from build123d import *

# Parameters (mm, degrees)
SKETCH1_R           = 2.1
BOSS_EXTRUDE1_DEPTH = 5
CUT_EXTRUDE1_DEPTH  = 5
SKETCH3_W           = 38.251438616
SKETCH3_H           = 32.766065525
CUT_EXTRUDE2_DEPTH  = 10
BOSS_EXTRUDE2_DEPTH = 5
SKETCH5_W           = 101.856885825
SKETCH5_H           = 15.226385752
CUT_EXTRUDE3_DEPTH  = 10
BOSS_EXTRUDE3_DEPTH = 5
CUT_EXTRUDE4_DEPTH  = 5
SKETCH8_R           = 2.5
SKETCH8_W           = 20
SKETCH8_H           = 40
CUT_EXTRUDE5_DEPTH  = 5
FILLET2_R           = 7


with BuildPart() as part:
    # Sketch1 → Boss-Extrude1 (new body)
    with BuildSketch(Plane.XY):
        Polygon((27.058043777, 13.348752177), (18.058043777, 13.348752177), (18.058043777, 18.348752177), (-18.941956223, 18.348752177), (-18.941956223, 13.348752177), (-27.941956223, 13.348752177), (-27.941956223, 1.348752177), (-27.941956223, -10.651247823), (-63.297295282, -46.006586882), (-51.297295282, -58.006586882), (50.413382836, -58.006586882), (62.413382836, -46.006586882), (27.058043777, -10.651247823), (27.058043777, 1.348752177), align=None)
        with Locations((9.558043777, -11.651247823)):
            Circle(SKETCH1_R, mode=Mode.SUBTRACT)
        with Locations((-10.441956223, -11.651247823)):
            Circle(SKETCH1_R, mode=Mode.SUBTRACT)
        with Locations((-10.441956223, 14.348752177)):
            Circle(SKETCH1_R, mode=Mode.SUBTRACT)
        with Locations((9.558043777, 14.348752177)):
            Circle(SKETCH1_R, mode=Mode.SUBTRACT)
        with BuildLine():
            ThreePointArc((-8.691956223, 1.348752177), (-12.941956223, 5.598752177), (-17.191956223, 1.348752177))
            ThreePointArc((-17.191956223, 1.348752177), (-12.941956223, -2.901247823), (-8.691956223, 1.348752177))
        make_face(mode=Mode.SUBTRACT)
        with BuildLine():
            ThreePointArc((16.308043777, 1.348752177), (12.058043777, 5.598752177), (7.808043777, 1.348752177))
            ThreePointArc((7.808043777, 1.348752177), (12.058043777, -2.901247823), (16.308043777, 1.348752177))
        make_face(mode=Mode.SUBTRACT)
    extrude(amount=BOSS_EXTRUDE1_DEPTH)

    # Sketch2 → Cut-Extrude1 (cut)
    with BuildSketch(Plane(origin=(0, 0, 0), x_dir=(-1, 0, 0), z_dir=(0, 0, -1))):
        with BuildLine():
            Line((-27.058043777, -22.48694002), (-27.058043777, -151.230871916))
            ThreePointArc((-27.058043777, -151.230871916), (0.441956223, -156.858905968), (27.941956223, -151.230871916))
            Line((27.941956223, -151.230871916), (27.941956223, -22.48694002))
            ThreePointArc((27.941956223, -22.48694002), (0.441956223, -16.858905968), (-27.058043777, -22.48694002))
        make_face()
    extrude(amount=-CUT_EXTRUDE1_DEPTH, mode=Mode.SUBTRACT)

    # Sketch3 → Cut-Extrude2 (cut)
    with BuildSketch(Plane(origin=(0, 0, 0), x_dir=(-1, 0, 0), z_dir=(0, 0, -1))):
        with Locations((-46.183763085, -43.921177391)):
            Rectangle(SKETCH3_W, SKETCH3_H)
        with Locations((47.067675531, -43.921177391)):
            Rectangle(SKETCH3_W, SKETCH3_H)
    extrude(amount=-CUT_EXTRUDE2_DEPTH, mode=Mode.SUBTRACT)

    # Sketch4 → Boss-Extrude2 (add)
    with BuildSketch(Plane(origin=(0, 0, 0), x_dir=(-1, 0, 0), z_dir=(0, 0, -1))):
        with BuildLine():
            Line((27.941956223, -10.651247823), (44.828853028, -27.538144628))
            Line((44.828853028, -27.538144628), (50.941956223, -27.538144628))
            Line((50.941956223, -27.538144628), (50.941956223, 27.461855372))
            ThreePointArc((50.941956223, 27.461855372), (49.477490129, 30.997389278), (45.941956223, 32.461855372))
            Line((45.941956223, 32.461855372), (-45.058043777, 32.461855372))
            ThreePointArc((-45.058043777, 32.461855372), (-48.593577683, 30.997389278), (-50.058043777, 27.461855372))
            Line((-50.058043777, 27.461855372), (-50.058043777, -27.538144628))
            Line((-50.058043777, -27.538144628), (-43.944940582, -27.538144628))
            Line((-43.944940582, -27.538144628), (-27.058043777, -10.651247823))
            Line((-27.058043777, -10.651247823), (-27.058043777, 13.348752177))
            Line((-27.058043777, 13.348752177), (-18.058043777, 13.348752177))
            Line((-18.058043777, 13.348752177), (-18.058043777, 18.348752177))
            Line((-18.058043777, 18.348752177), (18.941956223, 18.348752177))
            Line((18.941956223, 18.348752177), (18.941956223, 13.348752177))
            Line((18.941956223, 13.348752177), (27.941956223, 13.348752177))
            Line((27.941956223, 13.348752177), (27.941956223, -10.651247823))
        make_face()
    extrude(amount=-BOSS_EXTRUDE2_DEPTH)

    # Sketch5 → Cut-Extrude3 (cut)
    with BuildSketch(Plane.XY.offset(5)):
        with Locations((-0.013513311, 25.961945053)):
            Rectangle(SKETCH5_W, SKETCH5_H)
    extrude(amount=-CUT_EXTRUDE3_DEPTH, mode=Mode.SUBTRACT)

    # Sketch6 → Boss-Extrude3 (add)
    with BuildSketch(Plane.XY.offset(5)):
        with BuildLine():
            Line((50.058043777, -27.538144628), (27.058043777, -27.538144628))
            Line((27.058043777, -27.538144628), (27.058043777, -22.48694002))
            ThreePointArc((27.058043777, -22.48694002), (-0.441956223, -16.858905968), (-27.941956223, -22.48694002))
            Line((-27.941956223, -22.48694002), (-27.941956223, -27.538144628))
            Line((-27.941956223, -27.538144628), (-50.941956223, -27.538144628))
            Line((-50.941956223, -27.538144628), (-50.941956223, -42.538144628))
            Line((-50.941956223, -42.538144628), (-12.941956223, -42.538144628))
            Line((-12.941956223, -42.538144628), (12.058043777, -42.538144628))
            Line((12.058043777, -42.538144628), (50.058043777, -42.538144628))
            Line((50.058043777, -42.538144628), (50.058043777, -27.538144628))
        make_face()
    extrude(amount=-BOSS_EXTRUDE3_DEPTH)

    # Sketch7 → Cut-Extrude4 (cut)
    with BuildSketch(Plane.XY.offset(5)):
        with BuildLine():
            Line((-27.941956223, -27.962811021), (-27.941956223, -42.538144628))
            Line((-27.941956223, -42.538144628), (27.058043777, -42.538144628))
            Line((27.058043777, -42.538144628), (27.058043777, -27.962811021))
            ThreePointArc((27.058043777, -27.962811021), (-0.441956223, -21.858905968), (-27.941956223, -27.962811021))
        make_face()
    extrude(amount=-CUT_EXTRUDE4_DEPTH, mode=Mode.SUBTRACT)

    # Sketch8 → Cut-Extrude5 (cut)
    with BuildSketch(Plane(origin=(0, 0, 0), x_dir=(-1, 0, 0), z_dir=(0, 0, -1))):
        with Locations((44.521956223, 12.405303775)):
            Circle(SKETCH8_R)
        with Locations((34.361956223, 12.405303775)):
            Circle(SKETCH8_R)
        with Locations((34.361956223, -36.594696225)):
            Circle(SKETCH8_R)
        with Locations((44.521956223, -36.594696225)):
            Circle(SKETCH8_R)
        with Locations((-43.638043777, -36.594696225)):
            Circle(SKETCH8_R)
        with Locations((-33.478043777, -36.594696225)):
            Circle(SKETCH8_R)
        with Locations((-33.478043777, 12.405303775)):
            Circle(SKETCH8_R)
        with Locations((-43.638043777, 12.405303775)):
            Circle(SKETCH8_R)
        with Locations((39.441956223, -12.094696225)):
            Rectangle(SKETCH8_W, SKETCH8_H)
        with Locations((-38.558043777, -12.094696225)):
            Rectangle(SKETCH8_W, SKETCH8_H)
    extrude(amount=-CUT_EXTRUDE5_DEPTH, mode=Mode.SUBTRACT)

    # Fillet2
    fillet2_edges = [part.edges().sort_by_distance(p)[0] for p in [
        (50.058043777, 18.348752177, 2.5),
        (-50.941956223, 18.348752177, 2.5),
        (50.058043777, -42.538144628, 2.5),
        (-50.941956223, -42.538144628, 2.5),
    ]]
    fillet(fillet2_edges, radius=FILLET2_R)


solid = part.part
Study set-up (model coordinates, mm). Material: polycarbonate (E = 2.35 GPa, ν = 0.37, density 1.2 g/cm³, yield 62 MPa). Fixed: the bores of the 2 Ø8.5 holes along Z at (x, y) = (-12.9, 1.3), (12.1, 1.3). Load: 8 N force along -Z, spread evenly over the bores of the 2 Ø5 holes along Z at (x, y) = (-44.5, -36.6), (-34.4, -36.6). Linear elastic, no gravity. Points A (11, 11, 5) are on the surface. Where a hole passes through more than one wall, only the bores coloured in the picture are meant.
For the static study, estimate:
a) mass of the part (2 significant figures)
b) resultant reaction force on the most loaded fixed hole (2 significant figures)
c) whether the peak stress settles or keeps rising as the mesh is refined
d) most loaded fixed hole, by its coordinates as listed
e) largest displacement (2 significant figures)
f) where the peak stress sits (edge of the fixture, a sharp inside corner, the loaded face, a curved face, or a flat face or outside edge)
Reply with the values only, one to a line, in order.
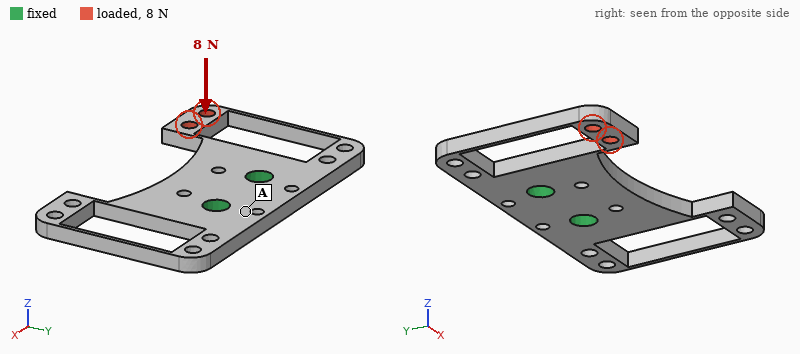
19 g
11 N
keeps rising
(-12.9, 1.3)
1.4 mm
a sharp inside corner
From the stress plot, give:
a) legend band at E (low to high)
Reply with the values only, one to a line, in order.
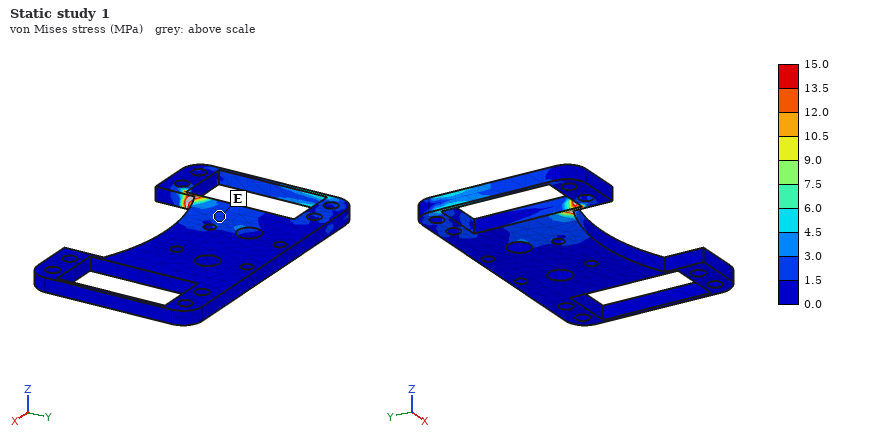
1.5 to 3.0 MPa
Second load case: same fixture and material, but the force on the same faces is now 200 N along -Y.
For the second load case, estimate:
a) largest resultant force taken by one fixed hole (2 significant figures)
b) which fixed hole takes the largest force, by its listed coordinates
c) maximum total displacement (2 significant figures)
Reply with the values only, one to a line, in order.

330 N
(-12.9, 1.3)
1.2 mm
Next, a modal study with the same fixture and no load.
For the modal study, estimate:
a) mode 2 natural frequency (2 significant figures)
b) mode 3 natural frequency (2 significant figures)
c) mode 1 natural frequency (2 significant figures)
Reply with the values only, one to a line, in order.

400 Hz
930 Hz
400 Hz
